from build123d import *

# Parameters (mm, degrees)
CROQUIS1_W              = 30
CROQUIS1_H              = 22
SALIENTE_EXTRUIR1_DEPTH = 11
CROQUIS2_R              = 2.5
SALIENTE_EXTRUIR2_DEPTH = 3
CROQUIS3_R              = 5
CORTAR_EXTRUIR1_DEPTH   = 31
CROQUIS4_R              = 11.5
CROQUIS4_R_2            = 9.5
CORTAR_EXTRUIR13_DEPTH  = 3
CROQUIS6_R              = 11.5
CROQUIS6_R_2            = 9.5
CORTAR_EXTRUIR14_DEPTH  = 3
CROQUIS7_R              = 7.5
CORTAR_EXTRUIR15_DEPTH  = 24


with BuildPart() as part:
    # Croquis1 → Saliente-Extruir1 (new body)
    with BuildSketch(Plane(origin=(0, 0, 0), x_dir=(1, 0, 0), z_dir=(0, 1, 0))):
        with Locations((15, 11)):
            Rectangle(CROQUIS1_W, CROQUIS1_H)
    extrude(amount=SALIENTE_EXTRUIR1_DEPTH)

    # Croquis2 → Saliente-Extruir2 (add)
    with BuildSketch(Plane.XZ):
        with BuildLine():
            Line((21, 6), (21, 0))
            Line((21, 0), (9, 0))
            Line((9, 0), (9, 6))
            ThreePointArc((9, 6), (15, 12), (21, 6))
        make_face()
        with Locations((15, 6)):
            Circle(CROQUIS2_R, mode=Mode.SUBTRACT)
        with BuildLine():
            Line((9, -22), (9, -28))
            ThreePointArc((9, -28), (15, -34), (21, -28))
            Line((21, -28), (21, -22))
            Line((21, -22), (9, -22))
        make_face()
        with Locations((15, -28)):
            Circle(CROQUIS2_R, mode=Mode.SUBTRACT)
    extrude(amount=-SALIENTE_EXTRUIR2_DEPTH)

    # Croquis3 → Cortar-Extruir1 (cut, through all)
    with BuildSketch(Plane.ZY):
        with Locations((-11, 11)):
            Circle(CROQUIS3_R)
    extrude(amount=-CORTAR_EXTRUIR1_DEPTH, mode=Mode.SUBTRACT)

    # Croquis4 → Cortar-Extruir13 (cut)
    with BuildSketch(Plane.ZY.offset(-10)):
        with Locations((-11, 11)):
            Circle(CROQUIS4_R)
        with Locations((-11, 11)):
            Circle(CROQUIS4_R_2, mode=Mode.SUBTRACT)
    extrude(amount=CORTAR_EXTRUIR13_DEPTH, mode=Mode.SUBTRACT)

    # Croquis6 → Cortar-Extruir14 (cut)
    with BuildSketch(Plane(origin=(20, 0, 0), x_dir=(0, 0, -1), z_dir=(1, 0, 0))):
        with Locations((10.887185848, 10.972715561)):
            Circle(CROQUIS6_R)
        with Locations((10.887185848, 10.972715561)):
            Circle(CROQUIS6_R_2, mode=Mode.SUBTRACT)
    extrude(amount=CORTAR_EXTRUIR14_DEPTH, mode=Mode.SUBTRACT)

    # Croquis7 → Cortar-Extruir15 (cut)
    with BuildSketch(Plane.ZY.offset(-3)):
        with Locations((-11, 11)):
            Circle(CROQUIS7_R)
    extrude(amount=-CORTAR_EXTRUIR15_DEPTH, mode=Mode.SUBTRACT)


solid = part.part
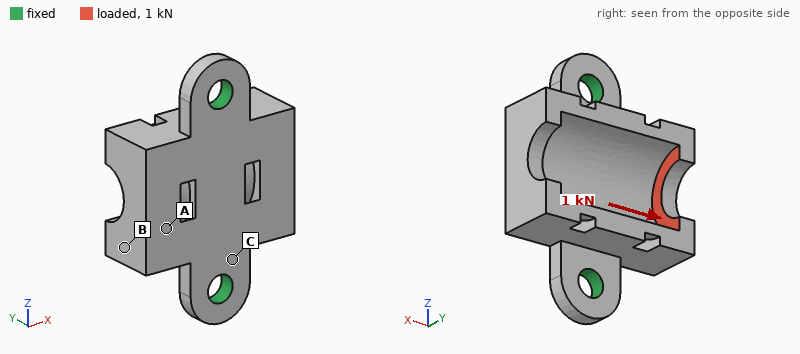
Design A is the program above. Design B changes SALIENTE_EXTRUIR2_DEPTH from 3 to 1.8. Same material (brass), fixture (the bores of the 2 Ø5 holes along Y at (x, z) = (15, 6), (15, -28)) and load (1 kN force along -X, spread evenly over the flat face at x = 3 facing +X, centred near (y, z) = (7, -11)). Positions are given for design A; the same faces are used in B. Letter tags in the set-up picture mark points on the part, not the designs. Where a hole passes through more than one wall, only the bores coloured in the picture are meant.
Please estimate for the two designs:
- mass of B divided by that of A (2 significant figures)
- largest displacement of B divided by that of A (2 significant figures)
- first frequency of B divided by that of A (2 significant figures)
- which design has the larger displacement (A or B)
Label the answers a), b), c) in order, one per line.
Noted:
a) 0.95
b) 3.0
c) 0.57
d) B
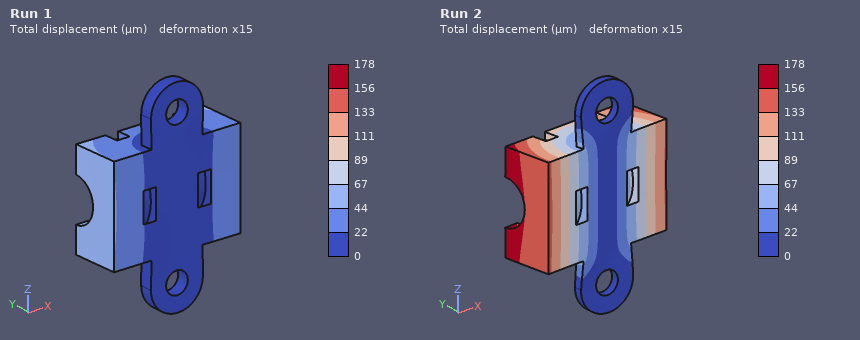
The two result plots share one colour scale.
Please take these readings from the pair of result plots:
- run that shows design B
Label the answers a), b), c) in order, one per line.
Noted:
a) Run 2
